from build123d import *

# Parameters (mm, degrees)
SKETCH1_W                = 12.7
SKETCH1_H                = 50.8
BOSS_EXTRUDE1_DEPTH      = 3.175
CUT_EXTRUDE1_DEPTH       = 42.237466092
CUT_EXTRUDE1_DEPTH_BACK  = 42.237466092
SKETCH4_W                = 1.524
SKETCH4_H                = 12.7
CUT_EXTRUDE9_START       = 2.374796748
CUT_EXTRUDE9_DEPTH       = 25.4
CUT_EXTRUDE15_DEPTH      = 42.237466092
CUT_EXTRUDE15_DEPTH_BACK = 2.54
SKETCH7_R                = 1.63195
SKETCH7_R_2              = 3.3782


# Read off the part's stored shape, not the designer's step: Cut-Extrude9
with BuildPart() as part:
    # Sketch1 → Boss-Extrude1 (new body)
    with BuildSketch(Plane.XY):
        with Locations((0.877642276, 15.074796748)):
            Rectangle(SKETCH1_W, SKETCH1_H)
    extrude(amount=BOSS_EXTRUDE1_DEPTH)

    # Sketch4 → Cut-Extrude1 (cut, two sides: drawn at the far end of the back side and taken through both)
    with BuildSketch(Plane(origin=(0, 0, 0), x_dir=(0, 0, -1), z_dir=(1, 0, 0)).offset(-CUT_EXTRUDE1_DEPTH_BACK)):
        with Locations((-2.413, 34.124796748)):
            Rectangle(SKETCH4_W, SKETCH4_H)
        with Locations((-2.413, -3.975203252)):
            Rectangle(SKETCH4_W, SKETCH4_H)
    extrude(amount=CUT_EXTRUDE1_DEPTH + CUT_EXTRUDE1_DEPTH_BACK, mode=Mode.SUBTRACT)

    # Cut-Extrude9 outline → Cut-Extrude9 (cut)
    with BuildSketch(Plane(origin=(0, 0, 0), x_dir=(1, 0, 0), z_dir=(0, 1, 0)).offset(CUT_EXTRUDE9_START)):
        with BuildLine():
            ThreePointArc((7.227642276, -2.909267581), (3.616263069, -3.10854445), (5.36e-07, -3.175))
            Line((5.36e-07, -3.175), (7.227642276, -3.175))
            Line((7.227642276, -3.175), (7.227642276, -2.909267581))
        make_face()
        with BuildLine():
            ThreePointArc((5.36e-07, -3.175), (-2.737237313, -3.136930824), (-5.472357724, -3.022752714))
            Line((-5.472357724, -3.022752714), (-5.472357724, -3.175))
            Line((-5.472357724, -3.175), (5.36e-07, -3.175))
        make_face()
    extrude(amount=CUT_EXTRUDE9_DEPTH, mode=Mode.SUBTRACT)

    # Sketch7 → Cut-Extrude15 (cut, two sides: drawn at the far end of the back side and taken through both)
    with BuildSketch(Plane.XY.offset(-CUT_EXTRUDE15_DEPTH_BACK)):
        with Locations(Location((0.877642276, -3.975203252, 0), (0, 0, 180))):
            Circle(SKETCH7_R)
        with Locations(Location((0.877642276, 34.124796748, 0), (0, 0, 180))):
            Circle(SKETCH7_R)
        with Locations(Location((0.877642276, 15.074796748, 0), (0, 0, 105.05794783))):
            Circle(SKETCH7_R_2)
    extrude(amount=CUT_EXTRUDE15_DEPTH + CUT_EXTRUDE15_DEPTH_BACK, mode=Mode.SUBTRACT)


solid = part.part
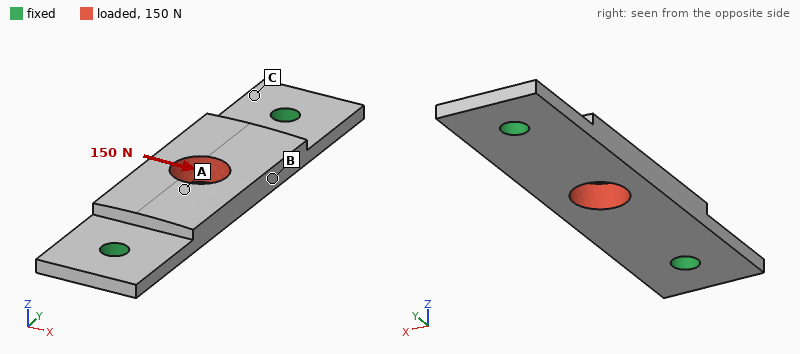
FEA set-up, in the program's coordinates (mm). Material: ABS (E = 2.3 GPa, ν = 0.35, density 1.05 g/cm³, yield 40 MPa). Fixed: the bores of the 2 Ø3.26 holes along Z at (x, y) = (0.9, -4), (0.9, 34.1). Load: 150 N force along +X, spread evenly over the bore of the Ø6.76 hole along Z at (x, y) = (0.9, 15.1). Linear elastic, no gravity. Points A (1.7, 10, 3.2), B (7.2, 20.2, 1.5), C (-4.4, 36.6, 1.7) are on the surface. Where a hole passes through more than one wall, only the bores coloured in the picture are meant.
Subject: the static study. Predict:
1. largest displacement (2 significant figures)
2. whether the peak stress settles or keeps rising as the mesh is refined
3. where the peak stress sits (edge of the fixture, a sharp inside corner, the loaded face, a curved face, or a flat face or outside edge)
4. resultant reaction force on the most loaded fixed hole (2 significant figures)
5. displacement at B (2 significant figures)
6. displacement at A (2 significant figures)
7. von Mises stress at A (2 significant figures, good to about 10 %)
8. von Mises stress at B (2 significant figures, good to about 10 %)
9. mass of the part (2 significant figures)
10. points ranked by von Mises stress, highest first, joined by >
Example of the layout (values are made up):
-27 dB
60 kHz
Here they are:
0.21 mm
keeps rising
edge of the fixture
75 N
0.17 mm
0.17 mm
4.7 MPa
9.2 MPa
1.5 g
B > A > C
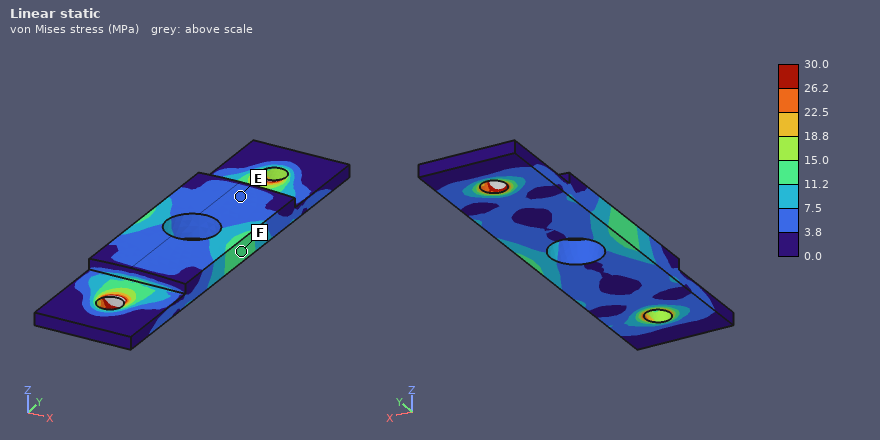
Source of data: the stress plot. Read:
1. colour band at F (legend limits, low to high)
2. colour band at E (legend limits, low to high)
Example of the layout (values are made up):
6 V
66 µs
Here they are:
11.2 to 15.0 MPa
3.8 to 7.5 MPa
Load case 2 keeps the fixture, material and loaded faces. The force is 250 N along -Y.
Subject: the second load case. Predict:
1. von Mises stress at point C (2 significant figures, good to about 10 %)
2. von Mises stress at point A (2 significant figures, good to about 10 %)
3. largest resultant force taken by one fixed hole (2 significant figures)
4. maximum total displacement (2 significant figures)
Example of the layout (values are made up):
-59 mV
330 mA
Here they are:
1.6 MPa
3.3 MPa
130 N
46 µm
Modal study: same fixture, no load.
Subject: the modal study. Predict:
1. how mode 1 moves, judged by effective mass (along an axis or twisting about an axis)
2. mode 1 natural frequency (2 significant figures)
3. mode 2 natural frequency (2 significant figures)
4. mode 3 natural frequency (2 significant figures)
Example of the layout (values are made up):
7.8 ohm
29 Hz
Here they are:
along Z
2300 Hz
3200 Hz
6000 Hz
